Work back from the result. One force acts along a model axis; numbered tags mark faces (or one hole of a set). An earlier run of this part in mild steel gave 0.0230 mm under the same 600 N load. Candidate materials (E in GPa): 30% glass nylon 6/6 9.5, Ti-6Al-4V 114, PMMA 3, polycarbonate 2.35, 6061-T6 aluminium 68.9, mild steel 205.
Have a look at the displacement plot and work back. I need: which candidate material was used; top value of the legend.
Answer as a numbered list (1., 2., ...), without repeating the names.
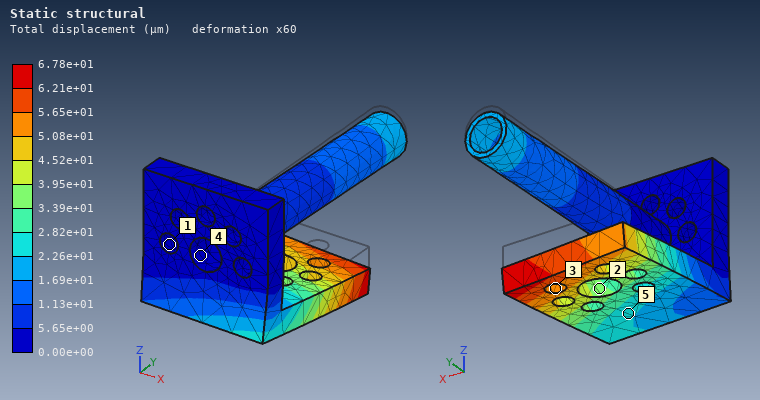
1. 6061-T6 aluminium
2. 6.78e+01 µm
